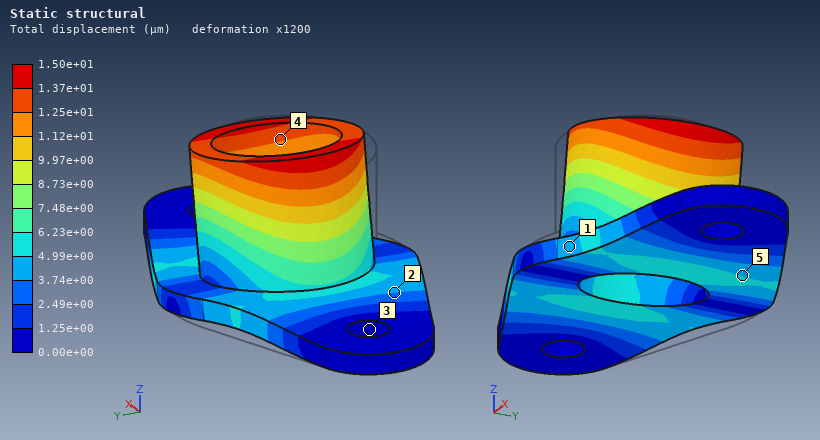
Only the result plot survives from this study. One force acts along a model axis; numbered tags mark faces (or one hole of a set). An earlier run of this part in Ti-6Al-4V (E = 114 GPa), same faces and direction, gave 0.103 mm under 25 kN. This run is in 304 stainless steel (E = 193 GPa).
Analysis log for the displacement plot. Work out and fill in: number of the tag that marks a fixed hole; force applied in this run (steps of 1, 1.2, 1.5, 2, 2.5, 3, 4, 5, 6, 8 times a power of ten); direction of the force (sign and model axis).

3
6 kN
+X
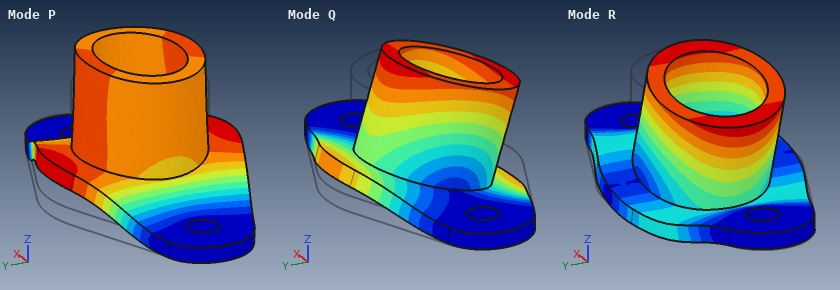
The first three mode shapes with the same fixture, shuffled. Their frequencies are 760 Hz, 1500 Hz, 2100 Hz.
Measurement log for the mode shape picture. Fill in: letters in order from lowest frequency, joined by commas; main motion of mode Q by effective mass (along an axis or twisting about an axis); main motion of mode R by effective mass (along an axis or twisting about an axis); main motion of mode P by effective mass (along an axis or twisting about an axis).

Q, P, R
along Y
along X
along Z
